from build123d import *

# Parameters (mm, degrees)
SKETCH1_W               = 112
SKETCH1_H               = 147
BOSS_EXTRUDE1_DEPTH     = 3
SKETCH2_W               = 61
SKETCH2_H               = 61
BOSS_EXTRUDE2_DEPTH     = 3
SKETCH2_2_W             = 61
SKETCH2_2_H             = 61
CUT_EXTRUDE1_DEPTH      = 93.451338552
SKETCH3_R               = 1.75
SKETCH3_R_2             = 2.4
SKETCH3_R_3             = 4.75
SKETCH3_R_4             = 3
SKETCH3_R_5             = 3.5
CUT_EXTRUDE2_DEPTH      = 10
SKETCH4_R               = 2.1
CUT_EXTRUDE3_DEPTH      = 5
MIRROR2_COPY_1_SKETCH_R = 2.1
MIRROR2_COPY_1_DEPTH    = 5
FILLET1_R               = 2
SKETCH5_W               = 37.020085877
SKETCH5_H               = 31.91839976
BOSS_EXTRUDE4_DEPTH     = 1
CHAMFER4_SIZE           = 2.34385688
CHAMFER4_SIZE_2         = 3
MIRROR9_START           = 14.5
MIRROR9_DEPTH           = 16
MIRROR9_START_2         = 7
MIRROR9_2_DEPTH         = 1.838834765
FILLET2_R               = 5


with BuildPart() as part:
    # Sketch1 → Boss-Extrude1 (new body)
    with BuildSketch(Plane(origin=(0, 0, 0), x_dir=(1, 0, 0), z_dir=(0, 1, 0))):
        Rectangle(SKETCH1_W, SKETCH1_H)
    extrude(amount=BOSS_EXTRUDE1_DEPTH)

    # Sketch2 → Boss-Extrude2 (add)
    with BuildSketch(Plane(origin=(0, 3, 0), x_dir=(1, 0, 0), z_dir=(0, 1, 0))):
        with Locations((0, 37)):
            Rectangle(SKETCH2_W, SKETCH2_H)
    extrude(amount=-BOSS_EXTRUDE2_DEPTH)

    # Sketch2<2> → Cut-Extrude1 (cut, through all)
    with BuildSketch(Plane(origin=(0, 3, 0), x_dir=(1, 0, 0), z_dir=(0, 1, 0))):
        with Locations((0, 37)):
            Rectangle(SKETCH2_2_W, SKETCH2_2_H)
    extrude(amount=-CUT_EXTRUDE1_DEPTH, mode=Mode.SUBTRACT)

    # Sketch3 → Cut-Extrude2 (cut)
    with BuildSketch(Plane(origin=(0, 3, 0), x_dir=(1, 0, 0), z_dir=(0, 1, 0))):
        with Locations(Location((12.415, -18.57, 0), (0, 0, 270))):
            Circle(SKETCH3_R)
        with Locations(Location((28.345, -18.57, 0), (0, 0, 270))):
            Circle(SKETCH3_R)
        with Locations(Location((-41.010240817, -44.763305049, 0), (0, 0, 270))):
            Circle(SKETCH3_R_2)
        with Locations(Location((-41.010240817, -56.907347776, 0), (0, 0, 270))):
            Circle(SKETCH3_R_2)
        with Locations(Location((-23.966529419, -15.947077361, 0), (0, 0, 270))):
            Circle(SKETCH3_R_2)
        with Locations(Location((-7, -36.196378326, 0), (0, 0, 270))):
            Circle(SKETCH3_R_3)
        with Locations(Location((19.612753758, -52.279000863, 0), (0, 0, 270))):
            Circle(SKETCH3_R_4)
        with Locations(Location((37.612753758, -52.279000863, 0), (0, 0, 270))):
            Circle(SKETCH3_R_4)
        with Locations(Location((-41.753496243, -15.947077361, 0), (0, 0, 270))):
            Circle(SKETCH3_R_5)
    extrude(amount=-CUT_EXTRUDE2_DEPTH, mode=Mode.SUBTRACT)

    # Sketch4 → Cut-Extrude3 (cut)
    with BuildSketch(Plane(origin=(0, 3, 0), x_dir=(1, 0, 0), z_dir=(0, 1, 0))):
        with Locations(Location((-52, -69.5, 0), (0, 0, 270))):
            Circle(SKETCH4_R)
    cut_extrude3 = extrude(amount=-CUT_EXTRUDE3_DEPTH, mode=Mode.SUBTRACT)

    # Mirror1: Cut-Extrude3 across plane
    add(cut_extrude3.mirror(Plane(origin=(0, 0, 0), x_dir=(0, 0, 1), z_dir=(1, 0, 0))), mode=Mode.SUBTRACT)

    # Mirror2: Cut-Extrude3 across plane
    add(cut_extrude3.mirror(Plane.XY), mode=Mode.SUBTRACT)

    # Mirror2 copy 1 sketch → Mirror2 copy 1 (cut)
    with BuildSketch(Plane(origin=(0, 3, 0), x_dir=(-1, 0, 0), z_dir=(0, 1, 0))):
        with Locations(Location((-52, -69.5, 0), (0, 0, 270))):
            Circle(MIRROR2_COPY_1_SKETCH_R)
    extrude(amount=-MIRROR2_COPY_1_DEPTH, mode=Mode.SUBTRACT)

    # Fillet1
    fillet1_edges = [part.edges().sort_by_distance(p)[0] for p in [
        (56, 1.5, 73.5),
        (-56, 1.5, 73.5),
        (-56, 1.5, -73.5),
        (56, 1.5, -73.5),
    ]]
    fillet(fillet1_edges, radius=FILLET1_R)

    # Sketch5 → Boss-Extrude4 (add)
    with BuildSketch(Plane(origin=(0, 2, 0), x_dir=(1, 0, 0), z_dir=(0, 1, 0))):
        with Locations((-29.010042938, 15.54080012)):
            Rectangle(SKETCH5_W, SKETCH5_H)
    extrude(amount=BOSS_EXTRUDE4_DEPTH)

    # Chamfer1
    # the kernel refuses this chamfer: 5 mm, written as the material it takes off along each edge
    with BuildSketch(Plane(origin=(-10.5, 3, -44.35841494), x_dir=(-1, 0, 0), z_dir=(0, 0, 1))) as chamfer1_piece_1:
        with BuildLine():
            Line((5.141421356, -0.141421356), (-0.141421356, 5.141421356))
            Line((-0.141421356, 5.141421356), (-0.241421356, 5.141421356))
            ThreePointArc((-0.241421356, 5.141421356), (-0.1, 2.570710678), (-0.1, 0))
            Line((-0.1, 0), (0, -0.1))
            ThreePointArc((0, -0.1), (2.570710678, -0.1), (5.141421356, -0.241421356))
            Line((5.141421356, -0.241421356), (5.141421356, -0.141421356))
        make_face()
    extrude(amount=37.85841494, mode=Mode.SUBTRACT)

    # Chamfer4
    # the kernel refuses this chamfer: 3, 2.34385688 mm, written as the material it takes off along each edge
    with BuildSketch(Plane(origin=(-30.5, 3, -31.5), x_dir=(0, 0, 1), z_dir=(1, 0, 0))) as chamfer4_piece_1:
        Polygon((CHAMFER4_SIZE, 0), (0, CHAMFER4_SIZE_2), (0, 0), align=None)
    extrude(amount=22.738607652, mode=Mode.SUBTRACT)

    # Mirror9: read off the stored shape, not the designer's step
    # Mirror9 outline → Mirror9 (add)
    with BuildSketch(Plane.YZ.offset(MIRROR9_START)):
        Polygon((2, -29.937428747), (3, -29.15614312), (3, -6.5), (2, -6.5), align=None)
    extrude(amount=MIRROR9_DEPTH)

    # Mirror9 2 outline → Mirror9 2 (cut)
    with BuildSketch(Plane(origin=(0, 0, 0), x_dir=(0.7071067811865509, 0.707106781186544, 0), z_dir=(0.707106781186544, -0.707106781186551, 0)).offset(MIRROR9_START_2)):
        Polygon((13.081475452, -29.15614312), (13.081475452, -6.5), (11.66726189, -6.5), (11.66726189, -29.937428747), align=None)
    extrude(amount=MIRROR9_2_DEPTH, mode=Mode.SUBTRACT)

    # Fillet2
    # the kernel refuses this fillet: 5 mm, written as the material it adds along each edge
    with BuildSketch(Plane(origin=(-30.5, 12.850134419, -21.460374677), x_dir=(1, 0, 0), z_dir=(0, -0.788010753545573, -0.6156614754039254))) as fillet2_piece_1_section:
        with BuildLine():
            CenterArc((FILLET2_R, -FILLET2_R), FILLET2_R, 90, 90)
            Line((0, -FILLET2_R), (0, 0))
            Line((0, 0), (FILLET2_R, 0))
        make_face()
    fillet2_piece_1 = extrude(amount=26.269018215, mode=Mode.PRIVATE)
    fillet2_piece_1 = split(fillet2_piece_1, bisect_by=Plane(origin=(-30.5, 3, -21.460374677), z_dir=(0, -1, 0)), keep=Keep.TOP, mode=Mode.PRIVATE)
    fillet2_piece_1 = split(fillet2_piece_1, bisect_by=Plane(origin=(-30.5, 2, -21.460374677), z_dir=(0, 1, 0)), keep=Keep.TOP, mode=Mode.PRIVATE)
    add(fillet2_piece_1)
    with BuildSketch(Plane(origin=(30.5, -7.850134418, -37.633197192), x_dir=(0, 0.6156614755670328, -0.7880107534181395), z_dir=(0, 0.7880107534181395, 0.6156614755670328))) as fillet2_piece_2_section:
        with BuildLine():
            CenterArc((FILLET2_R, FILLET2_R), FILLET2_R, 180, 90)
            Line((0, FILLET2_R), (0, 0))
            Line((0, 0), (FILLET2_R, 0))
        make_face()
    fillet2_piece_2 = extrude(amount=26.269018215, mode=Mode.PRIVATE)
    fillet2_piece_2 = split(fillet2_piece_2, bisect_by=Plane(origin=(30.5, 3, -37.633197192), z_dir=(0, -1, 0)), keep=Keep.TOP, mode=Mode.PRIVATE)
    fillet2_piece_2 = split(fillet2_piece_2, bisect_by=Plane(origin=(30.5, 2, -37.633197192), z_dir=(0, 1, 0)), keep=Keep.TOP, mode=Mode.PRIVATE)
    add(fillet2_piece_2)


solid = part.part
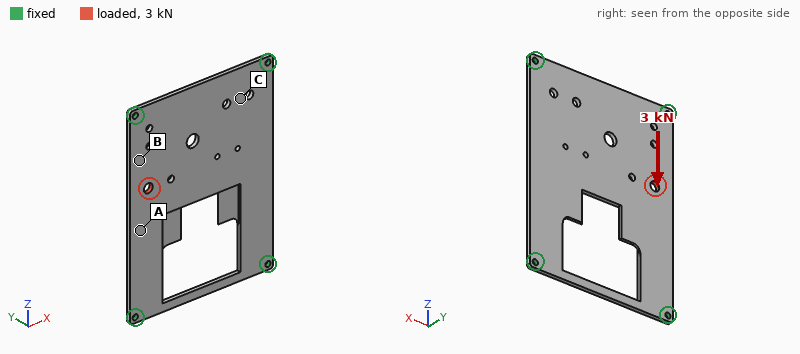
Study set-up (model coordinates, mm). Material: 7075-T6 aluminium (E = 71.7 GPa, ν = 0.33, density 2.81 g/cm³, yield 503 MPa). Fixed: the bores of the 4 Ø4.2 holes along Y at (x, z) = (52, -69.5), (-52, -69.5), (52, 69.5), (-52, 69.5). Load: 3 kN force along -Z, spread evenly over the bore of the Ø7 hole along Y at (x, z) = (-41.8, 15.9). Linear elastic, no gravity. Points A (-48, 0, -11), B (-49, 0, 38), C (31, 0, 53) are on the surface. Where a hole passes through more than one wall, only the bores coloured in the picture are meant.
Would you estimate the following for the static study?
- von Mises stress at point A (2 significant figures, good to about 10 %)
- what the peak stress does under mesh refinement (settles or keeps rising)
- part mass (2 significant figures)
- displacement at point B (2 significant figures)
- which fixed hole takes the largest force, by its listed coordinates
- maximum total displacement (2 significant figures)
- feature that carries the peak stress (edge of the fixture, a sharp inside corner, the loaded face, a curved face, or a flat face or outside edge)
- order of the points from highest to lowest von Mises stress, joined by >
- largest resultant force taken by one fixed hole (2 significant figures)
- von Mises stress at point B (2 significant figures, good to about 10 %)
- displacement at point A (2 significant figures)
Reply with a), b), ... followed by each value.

a) 17 MPa
b) keeps rising
c) 110 g
d) 17 µm
e) (-52, 69.5)
f) 26 µm
g) edge of the fixture
h) B > A > C
i) 1.7 kN
j) 28 MPa
k) 21 µm
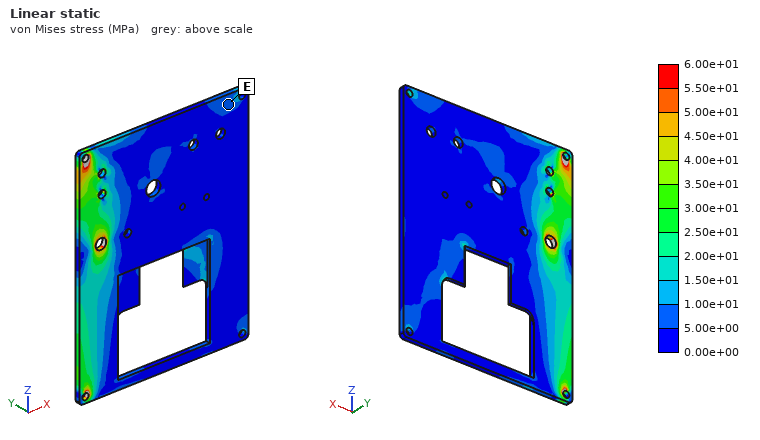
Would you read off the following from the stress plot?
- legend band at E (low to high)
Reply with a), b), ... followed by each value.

a) 5.00e+00 to 1.00e+01 MPa
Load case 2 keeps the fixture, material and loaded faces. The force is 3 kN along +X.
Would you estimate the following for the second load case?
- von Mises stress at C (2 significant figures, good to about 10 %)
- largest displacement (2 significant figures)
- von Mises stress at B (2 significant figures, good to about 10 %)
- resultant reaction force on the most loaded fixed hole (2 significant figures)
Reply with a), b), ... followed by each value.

a) 26 MPa
b) 48 µm
c) 12 MPa
d) 1.8 kN
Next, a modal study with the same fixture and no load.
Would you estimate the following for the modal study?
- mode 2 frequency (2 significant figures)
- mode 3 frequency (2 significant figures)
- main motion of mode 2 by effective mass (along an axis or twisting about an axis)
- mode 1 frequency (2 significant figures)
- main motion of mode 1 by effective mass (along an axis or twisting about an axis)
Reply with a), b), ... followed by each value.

a) 920 Hz
b) 1300 Hz
c) twisting about Z
d) 570 Hz
e) along Y
